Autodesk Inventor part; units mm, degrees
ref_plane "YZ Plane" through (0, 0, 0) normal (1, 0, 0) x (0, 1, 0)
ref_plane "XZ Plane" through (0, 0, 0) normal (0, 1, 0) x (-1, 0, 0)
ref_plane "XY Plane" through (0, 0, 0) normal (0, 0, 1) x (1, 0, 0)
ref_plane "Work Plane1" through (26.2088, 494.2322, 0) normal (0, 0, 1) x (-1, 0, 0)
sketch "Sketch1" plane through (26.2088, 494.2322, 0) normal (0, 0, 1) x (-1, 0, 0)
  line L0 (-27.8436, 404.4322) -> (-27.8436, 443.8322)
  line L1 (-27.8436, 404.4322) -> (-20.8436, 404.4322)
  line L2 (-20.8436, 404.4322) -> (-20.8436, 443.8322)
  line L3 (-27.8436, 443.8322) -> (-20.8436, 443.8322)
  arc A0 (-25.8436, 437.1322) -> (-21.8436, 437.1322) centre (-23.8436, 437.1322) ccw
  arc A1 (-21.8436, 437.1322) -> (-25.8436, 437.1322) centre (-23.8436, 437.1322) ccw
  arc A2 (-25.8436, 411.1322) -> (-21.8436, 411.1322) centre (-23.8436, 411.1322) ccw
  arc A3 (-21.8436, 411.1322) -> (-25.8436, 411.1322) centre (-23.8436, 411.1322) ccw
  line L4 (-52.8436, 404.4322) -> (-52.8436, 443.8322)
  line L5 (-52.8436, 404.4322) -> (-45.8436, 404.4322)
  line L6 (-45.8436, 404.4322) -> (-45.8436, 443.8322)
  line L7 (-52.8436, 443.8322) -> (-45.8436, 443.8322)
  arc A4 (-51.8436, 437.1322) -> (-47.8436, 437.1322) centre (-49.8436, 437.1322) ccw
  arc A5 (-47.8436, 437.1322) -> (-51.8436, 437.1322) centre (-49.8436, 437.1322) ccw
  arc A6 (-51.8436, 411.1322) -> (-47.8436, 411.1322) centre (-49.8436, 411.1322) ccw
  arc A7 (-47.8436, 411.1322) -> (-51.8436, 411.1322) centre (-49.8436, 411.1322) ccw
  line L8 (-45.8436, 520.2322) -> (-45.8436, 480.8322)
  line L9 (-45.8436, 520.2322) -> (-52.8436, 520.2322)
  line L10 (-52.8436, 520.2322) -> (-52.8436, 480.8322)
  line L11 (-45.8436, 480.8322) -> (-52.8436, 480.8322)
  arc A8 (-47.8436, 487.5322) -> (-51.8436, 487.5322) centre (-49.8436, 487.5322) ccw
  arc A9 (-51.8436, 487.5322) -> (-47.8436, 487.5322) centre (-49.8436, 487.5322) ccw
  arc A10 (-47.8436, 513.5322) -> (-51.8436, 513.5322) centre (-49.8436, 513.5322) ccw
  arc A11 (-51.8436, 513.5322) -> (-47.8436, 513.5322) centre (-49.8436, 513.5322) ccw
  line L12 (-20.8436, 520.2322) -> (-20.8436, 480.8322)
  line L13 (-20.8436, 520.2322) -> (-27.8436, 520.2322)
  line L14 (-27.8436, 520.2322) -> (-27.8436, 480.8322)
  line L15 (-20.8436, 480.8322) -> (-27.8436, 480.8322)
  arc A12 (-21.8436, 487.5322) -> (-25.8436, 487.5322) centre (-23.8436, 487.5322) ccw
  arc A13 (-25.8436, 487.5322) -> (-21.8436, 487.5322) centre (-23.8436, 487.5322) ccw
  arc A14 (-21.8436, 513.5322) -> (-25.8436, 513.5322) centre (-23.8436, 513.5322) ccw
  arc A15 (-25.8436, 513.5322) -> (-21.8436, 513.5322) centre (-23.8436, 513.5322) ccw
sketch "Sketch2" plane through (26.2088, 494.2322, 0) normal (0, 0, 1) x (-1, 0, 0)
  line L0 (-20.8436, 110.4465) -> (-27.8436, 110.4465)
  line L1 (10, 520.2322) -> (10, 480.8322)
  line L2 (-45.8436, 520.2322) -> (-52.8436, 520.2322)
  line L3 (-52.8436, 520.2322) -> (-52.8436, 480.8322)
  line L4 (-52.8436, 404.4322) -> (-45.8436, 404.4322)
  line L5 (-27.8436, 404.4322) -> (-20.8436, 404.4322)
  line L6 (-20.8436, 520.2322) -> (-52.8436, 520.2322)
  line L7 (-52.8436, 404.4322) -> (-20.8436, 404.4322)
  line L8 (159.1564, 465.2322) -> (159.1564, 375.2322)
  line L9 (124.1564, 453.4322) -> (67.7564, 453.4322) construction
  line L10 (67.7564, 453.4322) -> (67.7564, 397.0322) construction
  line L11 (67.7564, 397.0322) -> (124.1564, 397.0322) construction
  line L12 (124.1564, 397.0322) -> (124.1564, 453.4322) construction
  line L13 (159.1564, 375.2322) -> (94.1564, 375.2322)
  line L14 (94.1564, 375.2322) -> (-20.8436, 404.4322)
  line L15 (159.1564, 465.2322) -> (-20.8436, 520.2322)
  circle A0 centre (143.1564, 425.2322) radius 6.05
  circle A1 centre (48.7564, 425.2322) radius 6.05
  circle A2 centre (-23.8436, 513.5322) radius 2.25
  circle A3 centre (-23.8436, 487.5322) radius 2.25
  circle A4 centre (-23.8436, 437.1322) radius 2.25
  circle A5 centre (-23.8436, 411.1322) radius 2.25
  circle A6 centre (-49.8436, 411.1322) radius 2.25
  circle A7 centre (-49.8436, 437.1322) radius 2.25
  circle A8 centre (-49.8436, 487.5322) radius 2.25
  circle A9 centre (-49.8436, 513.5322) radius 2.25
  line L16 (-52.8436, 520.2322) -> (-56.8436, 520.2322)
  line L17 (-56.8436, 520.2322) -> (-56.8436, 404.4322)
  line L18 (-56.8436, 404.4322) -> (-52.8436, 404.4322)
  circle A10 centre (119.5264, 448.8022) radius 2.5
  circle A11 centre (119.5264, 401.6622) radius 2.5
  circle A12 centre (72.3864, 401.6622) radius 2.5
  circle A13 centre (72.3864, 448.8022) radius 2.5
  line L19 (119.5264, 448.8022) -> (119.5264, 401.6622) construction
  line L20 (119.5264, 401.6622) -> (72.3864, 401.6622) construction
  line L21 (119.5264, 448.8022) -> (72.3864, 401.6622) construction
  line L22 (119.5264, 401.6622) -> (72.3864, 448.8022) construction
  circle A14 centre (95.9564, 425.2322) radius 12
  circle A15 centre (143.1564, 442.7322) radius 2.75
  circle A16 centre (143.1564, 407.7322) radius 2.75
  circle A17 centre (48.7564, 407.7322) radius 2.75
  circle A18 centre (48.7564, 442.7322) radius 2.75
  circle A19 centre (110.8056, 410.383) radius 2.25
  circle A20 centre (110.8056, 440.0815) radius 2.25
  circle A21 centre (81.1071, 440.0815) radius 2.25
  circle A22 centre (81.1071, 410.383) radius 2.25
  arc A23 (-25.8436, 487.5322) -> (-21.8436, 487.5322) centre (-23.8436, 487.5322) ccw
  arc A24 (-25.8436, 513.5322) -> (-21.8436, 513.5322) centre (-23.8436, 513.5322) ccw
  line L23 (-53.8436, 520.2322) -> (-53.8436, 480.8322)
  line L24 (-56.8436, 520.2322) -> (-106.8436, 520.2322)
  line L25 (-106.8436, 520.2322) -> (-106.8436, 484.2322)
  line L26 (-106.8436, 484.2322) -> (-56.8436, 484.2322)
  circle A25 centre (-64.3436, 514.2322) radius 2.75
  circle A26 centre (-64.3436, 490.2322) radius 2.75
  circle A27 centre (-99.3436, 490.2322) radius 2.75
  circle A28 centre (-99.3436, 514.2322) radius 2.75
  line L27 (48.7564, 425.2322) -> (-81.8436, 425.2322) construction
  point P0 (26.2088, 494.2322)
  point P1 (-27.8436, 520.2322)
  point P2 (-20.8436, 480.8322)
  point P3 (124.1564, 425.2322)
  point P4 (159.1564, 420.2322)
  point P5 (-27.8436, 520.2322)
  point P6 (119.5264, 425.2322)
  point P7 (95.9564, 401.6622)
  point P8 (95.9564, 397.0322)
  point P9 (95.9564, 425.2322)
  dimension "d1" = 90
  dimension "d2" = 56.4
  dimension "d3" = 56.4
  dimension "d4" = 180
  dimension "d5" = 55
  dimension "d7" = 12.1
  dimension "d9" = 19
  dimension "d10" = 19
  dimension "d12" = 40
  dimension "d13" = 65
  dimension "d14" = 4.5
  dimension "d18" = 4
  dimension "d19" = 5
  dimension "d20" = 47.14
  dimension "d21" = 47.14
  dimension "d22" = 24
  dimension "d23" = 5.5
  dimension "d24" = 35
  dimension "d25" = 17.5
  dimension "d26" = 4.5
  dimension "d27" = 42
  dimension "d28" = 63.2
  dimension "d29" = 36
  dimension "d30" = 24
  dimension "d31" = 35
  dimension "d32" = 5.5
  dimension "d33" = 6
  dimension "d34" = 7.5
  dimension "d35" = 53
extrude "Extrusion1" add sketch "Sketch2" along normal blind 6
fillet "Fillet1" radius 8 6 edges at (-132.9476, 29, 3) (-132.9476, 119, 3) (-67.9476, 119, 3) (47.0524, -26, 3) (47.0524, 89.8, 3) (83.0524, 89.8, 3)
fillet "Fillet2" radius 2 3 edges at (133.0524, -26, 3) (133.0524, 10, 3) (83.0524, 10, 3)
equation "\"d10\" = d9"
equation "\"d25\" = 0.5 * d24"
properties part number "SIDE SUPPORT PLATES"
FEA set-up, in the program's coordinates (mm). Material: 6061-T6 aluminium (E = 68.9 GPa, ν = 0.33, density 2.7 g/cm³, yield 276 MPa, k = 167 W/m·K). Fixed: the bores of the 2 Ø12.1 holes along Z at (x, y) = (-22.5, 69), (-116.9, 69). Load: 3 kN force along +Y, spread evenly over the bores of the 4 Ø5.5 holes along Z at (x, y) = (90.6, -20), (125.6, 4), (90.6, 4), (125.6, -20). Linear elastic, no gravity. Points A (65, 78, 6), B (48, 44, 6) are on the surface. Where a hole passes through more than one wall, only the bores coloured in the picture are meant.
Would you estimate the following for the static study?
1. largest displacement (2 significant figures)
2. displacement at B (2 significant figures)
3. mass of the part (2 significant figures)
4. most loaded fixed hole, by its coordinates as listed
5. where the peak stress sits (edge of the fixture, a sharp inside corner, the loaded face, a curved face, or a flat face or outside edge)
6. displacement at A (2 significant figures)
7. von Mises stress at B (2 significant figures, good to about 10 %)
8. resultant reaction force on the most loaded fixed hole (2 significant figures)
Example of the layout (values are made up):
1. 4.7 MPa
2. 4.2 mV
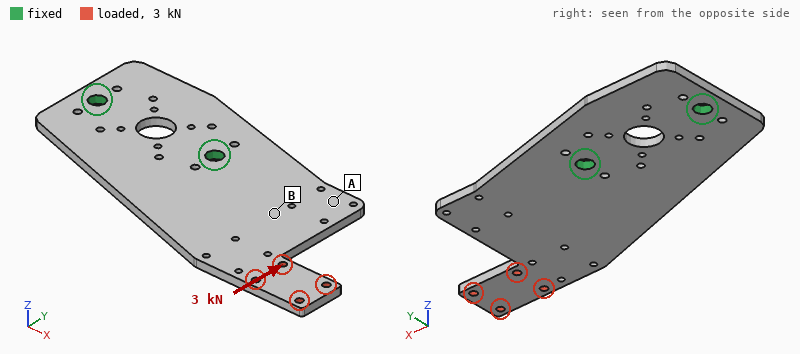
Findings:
1. 0.37 mm
2. 0.083 mm
3. 390 g
4. (-22.5, 69)
5. a curved face
6. 0.10 mm
7. 20 MPa
8. 6.7 kN
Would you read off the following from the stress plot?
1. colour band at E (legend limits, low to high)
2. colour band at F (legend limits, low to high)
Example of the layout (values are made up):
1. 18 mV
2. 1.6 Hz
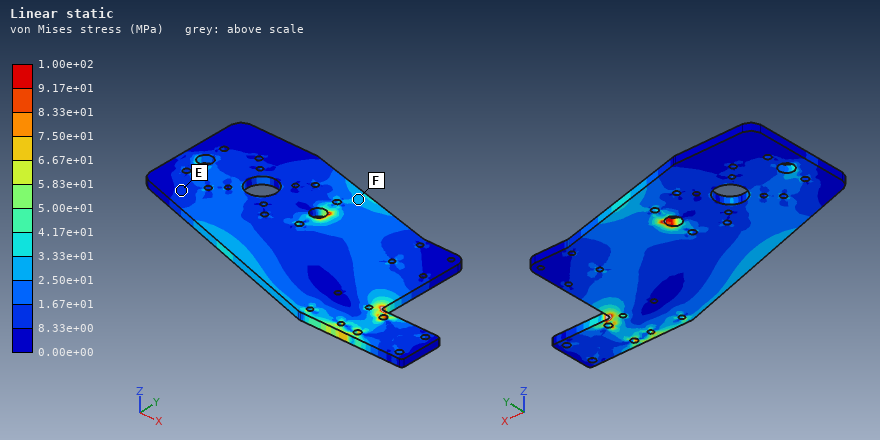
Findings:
1. 8.33e+00 to 1.67e+01 MPa
2. 2.50e+01 to 3.33e+01 MPa
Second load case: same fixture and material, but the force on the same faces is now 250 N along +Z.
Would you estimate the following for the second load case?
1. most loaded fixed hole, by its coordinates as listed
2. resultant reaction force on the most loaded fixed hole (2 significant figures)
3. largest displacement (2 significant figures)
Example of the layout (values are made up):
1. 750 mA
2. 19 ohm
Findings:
1. (-22.5, 69)
2. 380 N
3. 3.2 mm
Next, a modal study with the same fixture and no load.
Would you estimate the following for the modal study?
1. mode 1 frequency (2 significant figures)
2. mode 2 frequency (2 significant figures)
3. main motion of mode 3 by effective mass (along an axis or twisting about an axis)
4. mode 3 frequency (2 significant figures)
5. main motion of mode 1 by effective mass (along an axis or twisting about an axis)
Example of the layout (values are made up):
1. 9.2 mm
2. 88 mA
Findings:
1. 230 Hz
2. 700 Hz
3. along Z
4. 890 Hz
5. along Z
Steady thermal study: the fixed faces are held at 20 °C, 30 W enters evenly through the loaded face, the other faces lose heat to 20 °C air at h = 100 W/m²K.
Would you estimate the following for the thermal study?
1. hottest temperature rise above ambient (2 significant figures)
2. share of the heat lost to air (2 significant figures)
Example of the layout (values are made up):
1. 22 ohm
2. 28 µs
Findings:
1. 34 K
2. 86 %
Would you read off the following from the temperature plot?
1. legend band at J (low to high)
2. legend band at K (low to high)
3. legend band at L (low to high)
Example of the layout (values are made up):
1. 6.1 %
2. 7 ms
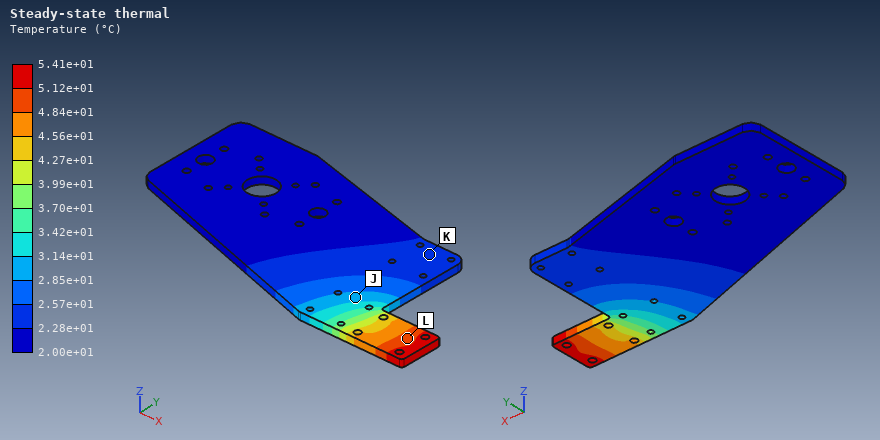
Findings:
1. 2.85e+01 to 3.14e+01 °C
2. 2.28e+01 to 2.57e+01 °C
3. 4.84e+01 to 5.12e+01 °C
